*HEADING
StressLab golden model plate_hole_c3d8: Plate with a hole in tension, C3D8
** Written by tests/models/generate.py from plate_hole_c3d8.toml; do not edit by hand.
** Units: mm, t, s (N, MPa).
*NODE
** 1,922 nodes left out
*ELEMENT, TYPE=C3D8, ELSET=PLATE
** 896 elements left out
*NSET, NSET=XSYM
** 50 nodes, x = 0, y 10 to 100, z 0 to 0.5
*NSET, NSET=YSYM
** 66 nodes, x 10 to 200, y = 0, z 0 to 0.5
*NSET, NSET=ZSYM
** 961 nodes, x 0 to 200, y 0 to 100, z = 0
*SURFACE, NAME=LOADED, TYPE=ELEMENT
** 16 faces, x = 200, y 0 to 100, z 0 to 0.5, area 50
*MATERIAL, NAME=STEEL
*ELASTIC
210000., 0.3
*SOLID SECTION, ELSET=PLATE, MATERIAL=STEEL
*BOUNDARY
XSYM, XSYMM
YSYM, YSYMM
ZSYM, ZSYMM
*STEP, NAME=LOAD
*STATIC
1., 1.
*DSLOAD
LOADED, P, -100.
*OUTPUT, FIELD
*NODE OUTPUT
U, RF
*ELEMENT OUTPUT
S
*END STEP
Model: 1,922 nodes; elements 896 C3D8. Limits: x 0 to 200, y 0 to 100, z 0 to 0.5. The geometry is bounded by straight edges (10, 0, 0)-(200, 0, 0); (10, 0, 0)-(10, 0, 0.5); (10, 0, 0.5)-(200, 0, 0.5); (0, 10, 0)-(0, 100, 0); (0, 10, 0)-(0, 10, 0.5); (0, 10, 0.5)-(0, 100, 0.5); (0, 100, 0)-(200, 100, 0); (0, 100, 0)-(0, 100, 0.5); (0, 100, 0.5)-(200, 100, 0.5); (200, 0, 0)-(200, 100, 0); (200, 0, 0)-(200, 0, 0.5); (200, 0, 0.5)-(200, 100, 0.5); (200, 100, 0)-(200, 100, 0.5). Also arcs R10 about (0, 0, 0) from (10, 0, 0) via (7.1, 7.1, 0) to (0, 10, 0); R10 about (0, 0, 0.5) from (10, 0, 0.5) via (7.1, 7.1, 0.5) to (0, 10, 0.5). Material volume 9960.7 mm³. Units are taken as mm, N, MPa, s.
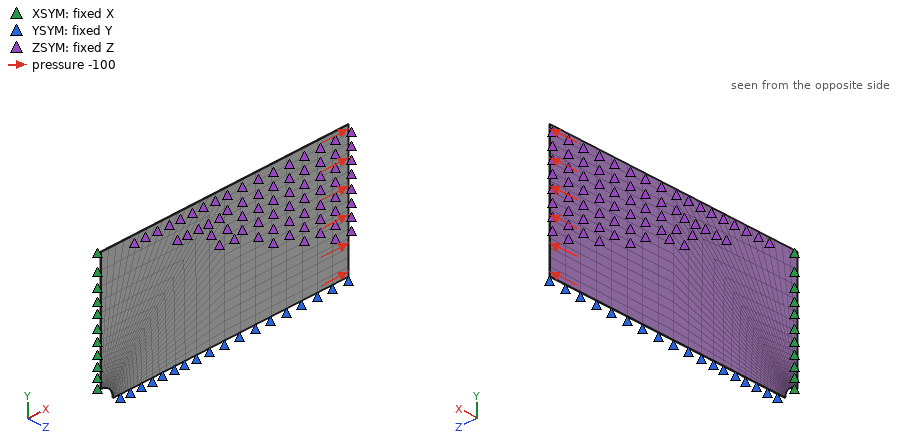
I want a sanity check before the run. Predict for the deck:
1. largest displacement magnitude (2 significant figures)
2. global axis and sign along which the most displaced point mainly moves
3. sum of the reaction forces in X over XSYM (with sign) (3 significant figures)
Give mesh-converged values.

0.097 mm
+X
-5000 N
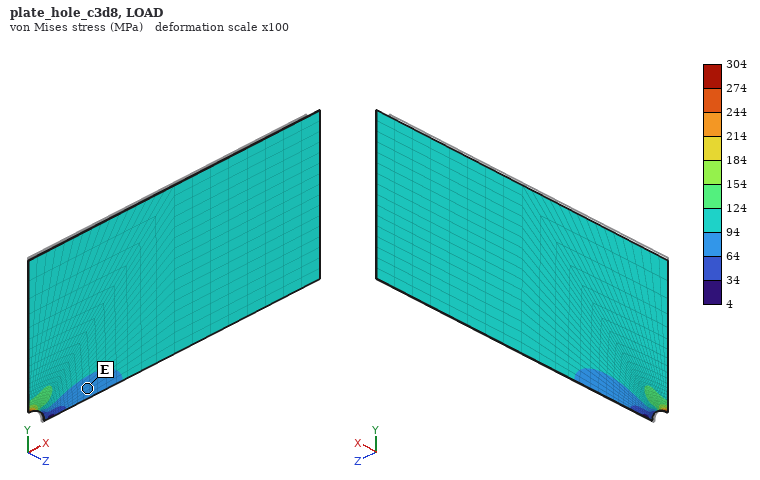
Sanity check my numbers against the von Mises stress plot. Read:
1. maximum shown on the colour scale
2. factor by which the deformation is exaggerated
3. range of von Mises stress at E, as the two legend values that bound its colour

304 MPa
100
64 to 94 MPa
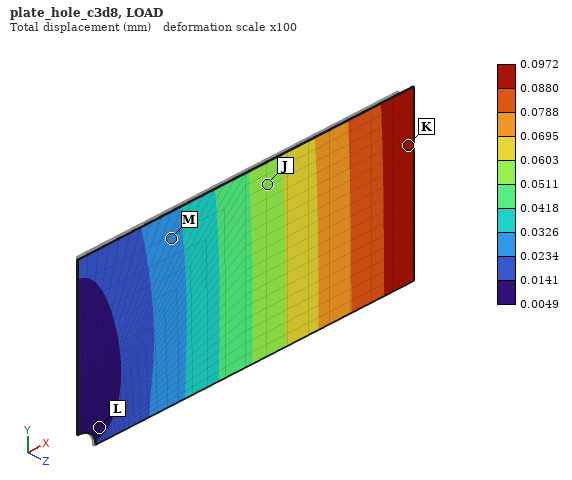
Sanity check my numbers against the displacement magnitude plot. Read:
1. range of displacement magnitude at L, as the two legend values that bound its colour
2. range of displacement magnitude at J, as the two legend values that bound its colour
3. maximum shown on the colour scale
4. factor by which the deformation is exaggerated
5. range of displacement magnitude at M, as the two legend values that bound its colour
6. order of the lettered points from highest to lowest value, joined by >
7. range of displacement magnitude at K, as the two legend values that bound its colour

0.0049 to 0.0141 mm
0.0511 to 0.0603 mm
0.0972 mm
100
0.0234 to 0.0326 mm
K > J > M > L
0.0880 to 0.0972 mm
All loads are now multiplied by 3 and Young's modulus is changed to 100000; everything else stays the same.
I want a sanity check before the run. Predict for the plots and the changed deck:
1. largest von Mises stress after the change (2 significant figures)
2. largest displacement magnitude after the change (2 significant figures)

910 MPa
0.61 mm
